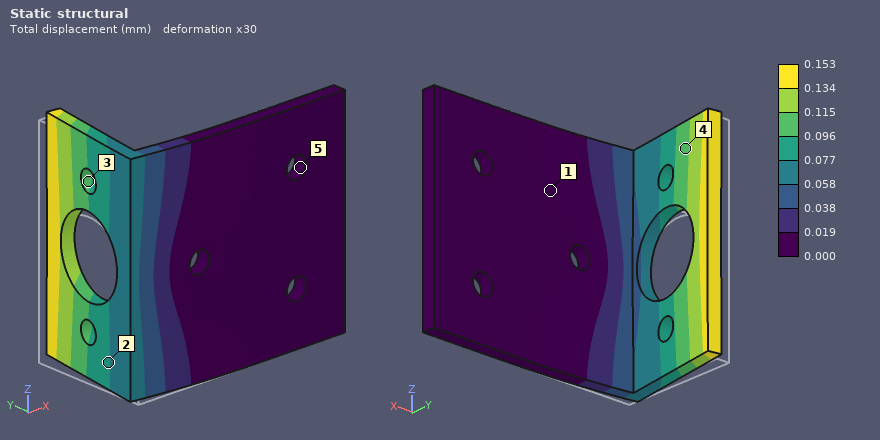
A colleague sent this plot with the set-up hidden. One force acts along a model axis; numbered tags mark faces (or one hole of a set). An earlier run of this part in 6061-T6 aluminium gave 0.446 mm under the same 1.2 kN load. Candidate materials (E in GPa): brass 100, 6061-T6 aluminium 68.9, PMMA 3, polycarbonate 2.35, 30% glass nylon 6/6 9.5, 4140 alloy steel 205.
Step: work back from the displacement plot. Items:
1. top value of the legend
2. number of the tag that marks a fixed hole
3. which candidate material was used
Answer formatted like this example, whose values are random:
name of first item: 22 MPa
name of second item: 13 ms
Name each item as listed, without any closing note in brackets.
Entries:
top value of the legend: 0.153 mm
number of the tag that marks a fixed hole: 5
which candidate material was used: 4140 alloy steel
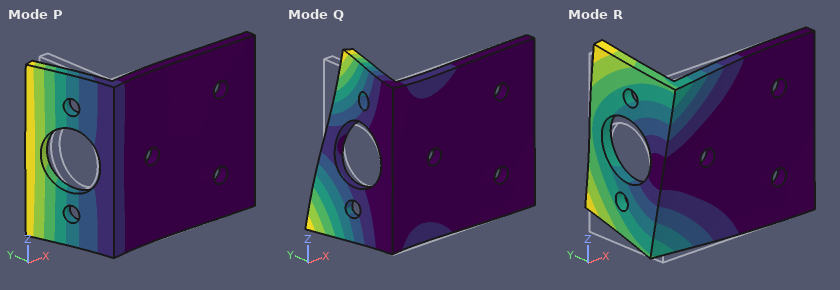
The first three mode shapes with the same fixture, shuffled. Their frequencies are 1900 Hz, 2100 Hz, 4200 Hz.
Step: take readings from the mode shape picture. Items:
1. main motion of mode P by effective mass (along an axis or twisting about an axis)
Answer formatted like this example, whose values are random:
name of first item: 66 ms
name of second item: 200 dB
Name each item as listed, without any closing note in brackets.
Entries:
main motion of mode P by effective mass: along X
